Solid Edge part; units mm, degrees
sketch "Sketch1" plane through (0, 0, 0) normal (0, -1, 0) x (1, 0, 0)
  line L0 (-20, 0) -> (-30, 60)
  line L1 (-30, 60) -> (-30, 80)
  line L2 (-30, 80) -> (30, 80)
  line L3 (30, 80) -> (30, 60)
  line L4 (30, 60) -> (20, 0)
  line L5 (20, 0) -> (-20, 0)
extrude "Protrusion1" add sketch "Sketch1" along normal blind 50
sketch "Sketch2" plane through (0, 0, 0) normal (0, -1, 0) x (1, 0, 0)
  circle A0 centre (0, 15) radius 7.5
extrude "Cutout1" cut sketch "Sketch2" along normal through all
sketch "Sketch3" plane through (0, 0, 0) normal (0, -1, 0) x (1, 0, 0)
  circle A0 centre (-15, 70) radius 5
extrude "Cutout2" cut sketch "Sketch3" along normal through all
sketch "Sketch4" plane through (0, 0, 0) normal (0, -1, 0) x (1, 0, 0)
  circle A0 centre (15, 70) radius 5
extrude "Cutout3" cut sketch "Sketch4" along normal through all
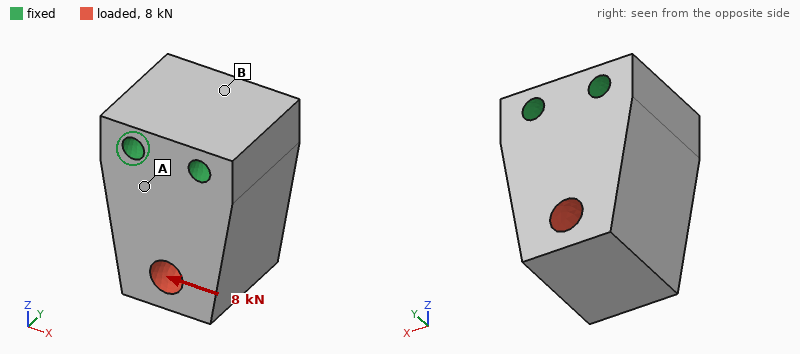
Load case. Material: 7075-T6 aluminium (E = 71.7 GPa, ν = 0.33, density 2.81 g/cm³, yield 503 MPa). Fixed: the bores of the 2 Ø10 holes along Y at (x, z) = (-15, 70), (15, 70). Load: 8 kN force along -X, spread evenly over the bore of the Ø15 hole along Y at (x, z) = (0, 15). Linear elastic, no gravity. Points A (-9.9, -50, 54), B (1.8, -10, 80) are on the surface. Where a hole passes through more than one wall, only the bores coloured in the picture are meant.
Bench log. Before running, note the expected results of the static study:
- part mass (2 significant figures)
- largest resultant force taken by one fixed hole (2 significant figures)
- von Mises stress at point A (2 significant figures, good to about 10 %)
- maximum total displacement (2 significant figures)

540 g
12 kN
8.2 MPa
23 µm
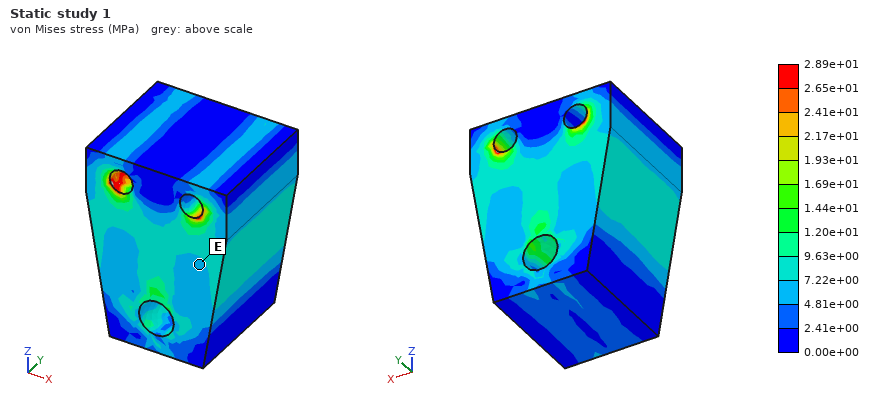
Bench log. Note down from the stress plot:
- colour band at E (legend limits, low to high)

4.81e+00 to 7.22e+00 MPa
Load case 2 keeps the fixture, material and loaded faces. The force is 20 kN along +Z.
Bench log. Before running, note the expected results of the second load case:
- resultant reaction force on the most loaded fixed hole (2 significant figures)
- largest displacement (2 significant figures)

10 kN
11 µm
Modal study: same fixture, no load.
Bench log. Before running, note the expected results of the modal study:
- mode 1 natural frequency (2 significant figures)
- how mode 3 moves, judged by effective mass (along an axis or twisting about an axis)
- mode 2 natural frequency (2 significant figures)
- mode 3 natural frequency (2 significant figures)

7400 Hz
twisting about Z
7600 Hz
12 kHz
